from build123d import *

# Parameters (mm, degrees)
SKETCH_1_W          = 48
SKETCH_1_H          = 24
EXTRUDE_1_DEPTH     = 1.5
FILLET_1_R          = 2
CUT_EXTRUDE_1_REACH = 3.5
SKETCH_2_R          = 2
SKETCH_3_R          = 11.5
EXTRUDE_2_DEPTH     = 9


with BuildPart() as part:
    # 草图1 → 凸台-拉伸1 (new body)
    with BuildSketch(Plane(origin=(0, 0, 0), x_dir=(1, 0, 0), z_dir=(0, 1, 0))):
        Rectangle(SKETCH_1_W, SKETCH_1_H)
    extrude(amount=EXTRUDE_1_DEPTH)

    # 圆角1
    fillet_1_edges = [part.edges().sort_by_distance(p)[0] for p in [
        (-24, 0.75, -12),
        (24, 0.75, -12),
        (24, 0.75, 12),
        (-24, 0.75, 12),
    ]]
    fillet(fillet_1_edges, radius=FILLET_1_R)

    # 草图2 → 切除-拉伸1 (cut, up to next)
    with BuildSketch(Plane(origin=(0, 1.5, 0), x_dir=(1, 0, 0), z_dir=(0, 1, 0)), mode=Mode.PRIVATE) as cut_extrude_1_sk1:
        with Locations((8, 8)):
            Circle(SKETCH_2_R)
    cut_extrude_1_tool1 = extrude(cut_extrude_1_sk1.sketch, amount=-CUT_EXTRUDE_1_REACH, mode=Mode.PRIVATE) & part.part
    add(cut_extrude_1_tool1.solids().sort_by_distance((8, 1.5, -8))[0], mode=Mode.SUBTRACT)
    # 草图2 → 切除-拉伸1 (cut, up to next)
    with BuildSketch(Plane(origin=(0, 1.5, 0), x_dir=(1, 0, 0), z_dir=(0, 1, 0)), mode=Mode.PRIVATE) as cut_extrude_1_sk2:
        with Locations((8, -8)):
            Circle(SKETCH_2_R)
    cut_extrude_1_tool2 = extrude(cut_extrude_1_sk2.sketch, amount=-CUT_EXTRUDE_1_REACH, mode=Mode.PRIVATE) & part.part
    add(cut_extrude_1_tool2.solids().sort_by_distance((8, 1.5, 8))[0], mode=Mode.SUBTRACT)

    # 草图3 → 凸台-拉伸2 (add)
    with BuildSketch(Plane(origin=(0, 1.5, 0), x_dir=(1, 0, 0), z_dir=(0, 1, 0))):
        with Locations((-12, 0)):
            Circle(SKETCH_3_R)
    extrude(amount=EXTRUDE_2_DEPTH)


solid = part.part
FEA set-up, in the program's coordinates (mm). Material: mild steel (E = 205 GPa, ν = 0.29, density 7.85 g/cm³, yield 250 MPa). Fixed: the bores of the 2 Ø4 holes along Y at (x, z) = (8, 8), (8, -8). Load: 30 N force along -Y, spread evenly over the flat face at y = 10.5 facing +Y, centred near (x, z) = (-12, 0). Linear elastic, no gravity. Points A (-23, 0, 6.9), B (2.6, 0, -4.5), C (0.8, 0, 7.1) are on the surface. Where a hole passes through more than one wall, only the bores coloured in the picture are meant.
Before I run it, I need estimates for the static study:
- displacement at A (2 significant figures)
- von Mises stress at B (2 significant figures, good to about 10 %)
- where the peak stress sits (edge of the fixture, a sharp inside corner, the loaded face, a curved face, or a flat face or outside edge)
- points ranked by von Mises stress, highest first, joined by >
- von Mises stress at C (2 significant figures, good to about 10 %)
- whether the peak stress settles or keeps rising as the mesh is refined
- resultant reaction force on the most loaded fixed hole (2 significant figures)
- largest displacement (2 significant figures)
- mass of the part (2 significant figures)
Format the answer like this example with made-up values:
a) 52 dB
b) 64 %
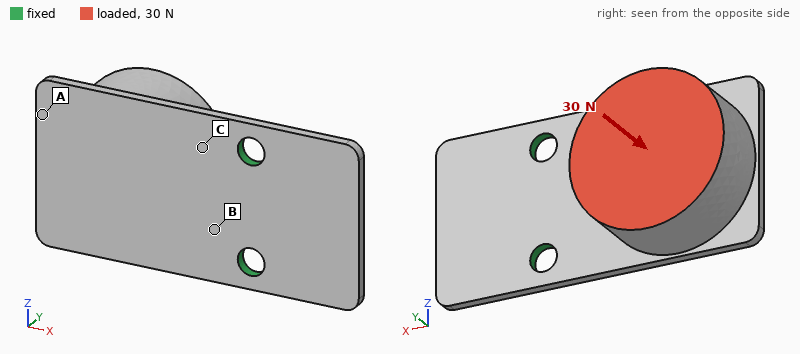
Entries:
a) 68 µm
b) 43 MPa
c) edge of the fixture
d) B > C > A
e) 36 MPa
f) keeps rising
g) 15 N
h) 74 µm
i) 43 g
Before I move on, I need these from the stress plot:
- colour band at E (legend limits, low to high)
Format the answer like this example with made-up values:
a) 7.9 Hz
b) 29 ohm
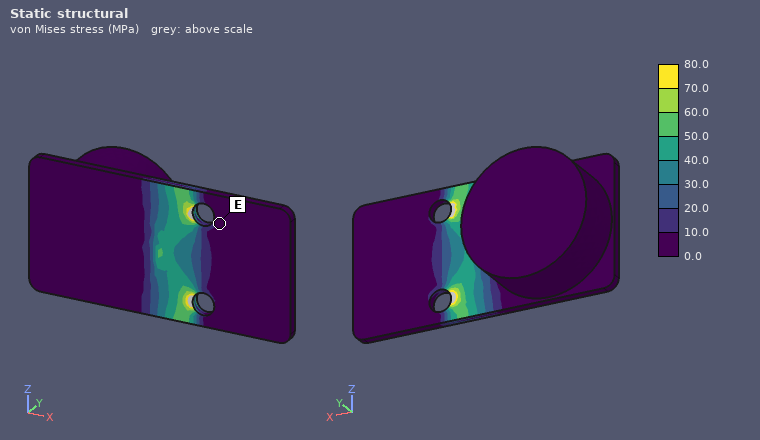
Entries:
a) 0.0 to 10.0 MPa
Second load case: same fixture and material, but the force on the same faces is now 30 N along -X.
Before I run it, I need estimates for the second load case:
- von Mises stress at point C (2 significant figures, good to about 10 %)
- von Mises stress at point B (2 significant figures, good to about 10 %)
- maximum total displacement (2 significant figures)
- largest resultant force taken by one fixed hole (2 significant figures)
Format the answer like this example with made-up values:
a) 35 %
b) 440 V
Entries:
a) 26 MPa
b) 28 MPa
c) 49 µm
d) 16 N
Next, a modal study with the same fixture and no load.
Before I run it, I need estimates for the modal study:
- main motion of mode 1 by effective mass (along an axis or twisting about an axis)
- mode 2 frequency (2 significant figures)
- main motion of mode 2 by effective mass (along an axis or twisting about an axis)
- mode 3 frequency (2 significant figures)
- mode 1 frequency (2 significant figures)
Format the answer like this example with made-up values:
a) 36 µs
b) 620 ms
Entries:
a) along Y
b) 3000 Hz
c) along Z
d) 5600 Hz
e) 650 Hz
